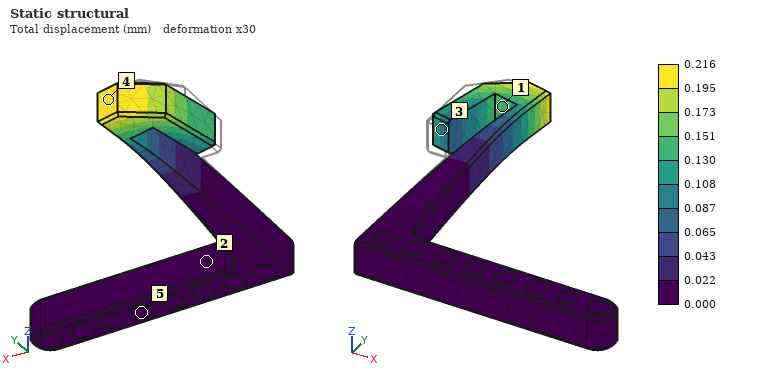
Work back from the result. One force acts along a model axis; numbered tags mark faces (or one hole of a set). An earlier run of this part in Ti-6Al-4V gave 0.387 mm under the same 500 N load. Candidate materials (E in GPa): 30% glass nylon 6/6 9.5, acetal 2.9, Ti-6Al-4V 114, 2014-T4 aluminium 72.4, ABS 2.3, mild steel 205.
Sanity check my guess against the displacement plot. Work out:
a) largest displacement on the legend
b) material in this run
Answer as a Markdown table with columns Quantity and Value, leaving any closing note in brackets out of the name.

| Quantity | Value |
|---|---|
| largest displacement on the legend | 0.216 mm |
| material in this run | mild steel |
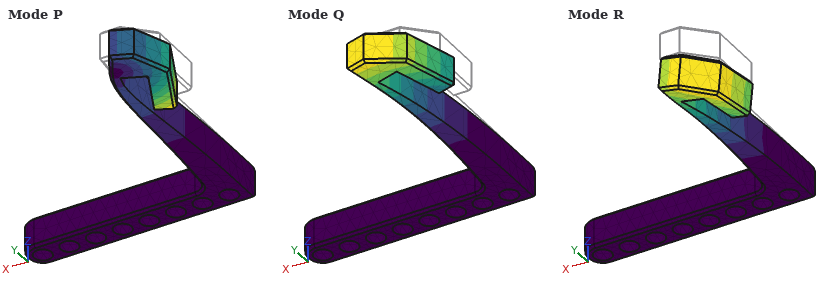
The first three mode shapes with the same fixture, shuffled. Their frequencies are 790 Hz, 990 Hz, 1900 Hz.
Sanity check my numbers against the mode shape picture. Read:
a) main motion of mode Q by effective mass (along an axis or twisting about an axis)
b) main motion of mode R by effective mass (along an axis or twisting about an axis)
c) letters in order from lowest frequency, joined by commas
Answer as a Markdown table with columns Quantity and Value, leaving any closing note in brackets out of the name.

| Quantity | Value |
|---|---|
| main motion of mode Q by effective mass | along X |
| main motion of mode R by effective mass | along Z |
| letters in order from lowest frequency, joined by commas | Q, R, P |
